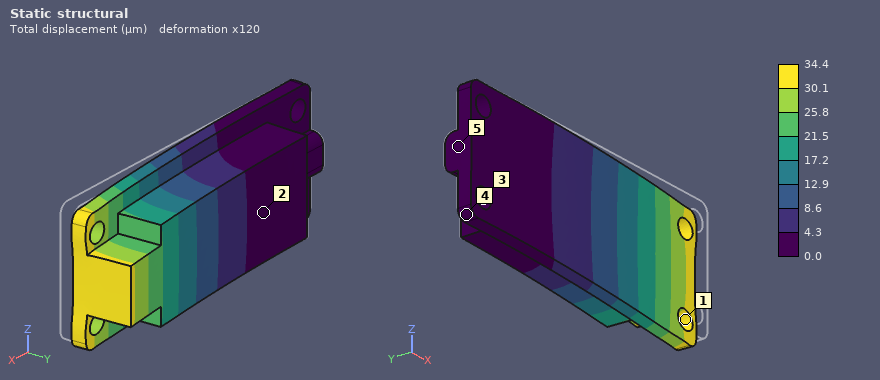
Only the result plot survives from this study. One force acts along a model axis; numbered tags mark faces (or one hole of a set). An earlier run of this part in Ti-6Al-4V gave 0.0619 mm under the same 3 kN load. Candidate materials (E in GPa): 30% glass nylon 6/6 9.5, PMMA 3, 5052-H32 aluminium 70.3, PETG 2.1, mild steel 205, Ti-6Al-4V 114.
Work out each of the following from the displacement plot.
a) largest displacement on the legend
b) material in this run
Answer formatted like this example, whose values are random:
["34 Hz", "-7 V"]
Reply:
["34.4 µm", "mild steel"]
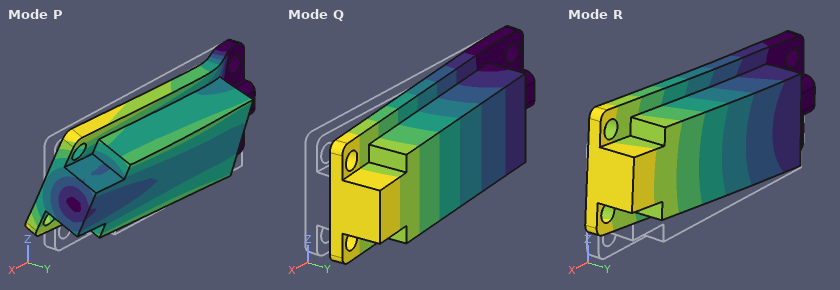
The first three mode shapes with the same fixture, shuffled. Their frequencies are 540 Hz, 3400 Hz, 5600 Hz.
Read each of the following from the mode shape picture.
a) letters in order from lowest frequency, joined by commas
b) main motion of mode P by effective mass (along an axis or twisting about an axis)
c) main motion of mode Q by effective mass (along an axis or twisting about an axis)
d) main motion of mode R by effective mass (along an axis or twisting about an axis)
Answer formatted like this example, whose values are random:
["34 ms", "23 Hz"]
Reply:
["Q, R, P", "twisting about X", "along Y", "along Z"]
